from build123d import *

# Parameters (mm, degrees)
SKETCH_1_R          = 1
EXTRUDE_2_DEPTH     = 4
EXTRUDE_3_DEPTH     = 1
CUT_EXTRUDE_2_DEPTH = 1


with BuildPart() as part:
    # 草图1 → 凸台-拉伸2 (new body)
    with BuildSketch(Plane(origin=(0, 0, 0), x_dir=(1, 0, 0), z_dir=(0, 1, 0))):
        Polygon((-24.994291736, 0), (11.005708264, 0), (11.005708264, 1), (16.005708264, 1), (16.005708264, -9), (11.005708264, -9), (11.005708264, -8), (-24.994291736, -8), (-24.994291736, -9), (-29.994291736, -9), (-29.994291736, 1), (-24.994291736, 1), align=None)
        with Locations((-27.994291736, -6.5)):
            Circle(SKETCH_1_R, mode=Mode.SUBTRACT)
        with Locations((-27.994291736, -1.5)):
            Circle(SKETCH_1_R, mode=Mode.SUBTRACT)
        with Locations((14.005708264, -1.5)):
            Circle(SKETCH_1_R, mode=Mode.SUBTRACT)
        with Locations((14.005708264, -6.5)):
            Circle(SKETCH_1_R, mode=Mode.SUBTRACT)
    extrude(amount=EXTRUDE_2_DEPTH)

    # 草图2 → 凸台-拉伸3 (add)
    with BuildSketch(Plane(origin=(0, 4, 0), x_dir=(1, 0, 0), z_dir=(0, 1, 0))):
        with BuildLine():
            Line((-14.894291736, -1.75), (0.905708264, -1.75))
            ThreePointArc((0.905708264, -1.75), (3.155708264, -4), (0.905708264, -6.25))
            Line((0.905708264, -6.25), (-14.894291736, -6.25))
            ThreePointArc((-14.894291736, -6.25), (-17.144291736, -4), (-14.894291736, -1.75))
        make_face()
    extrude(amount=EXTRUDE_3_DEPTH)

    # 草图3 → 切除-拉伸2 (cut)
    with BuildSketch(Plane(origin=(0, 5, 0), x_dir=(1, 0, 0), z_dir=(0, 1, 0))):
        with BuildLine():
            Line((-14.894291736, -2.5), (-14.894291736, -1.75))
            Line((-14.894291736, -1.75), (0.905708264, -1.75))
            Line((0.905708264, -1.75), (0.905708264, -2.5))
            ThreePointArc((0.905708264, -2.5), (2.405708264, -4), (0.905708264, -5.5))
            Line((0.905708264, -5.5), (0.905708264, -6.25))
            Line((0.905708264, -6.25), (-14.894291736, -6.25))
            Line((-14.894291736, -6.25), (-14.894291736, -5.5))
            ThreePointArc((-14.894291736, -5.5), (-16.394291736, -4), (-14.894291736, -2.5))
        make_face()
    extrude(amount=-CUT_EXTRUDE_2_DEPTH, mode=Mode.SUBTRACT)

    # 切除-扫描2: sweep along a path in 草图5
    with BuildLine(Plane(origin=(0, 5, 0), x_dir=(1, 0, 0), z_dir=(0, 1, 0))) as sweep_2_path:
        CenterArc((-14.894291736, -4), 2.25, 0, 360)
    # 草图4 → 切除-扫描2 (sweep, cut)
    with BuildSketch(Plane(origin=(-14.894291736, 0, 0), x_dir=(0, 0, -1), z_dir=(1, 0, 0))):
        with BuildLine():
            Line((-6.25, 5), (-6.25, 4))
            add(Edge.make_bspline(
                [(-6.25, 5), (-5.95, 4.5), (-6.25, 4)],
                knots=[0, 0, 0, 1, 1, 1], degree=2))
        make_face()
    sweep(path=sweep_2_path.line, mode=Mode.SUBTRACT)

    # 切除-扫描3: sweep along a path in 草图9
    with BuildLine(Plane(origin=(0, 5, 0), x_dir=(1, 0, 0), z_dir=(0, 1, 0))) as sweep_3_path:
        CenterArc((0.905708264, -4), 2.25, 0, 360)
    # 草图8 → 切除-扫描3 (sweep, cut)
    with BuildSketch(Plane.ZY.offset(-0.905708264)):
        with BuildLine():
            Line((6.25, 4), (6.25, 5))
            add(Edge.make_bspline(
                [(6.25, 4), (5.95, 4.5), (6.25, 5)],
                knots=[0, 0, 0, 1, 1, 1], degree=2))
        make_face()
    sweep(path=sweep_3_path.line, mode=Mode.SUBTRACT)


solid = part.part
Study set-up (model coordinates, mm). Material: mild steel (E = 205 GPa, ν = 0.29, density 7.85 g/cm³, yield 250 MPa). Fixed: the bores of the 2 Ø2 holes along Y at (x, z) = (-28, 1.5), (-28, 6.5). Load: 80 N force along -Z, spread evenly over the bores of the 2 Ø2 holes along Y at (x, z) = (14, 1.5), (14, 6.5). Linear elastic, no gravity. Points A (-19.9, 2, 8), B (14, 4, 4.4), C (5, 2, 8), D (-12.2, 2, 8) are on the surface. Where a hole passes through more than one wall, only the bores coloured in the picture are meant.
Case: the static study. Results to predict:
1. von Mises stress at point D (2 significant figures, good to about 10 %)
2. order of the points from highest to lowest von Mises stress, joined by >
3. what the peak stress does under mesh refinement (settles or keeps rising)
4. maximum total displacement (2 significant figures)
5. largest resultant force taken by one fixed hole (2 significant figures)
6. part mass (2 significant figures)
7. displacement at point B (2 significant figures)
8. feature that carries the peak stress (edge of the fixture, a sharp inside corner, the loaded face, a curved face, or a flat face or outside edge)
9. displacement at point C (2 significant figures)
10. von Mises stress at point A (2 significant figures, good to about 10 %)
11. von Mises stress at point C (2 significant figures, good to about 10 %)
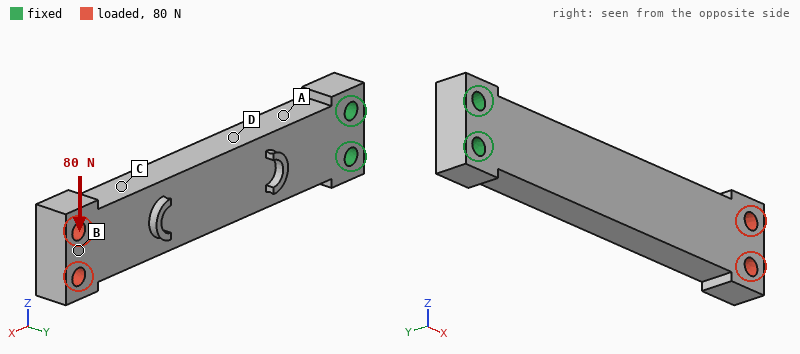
49 MPa
A > D > C > B
keeps rising
58 µm
550 N
12 g
54 µm
edge of the fixture
37 µm
63 MPa
17 MPa
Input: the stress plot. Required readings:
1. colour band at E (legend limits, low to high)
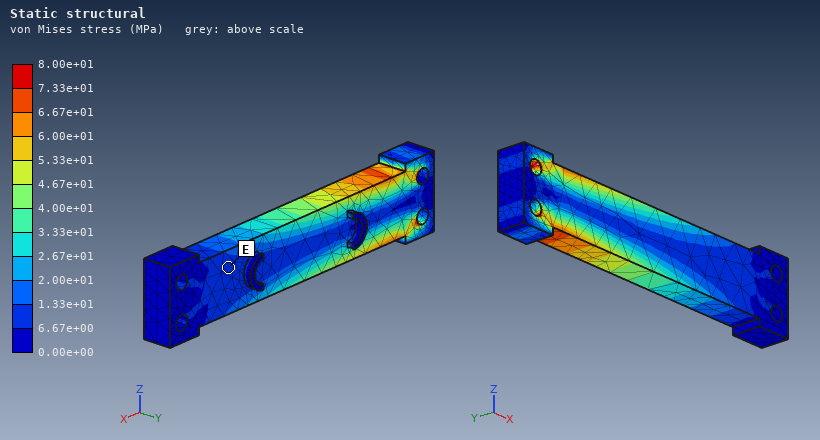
6.67e+00 to 1.33e+01 MPa
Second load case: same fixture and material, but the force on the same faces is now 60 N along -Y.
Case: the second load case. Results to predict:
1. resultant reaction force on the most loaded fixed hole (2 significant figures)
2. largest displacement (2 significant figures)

30 N
0.17 mm
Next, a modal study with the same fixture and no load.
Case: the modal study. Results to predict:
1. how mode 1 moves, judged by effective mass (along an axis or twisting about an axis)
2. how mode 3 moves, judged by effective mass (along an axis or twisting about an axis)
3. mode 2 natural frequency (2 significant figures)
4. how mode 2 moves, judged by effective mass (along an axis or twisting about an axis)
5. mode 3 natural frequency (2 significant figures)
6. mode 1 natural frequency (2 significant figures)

along Y
along Y
3400 Hz
along Z
10 kHz
1700 Hz
